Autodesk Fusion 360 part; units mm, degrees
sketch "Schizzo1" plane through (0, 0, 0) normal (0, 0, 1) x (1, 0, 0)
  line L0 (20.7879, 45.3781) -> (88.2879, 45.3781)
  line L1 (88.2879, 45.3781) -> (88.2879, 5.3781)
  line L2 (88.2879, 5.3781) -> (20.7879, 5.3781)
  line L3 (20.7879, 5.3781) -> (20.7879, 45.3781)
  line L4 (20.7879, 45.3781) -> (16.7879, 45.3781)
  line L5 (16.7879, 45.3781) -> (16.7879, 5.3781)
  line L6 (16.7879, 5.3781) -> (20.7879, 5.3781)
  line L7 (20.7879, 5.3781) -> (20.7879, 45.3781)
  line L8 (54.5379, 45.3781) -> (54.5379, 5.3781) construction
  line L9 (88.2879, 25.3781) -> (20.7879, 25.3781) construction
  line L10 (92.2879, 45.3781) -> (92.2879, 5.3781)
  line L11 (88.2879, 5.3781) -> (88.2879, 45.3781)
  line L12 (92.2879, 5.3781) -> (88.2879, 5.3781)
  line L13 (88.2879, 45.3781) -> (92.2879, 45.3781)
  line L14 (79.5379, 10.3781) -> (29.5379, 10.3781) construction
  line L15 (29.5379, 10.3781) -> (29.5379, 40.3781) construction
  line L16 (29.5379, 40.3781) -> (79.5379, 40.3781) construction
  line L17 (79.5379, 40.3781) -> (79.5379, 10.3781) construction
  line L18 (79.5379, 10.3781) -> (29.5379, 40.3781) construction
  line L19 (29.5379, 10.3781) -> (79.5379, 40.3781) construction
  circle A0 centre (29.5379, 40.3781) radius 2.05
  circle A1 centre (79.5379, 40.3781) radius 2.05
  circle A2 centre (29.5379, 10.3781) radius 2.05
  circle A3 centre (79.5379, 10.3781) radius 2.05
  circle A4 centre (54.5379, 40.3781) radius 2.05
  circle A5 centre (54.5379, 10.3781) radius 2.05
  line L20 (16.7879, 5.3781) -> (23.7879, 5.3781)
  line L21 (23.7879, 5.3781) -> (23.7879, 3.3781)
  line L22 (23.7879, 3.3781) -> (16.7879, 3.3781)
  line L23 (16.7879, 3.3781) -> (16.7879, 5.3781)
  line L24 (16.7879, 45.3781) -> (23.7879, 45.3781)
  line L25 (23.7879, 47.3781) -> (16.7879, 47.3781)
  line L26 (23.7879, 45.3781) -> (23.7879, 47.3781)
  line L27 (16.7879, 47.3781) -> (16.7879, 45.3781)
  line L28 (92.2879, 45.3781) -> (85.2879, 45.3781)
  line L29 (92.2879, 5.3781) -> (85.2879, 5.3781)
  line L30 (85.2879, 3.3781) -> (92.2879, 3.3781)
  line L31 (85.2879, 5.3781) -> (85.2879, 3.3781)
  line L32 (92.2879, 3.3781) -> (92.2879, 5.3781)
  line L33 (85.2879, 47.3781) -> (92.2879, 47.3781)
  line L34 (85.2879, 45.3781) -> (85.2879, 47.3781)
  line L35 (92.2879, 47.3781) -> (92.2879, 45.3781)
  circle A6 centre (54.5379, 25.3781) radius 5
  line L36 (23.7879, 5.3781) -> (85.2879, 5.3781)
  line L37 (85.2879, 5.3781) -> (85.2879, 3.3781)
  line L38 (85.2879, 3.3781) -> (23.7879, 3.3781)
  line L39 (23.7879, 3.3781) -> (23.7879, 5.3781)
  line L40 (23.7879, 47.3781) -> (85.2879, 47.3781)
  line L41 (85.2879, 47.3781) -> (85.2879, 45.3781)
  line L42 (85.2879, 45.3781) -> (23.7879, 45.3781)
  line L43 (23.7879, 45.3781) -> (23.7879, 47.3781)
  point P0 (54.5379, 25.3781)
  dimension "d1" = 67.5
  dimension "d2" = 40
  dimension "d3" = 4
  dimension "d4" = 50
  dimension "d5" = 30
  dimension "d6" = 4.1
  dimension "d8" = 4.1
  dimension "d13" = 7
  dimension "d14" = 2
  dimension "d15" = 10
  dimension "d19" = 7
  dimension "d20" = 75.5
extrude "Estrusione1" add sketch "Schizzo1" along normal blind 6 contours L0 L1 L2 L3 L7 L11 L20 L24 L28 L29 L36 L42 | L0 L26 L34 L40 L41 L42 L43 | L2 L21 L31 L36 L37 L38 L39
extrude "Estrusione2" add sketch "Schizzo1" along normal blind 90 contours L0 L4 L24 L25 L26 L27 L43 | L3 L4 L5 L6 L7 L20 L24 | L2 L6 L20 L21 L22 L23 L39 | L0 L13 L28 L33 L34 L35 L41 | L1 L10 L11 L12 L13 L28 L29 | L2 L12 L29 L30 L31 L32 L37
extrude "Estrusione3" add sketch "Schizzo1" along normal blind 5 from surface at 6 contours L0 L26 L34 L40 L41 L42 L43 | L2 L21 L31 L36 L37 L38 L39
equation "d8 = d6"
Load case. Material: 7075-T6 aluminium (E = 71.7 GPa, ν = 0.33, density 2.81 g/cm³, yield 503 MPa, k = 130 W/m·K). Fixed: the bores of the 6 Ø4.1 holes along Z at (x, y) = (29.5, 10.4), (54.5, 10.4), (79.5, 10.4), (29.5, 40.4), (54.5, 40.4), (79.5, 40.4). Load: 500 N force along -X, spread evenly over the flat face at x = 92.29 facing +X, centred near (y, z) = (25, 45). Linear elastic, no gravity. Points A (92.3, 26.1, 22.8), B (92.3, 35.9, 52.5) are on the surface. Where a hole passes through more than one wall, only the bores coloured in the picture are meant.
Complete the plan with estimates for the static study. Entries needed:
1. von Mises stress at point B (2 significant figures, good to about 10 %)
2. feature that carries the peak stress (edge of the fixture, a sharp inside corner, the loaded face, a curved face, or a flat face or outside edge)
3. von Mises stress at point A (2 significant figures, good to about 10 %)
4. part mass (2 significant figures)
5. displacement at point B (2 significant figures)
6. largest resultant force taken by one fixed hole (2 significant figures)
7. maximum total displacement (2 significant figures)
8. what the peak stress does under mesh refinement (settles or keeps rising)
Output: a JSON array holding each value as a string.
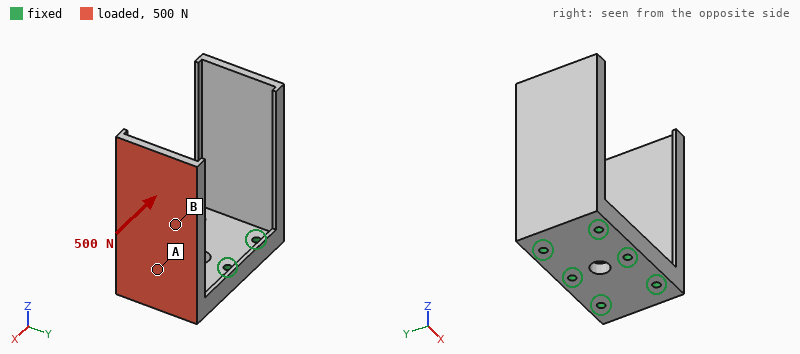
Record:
["25 MPa", "a sharp inside corner", "61 MPa", "150 g", "0.65 mm", "270 N", "1.5 mm", "keeps rising"]
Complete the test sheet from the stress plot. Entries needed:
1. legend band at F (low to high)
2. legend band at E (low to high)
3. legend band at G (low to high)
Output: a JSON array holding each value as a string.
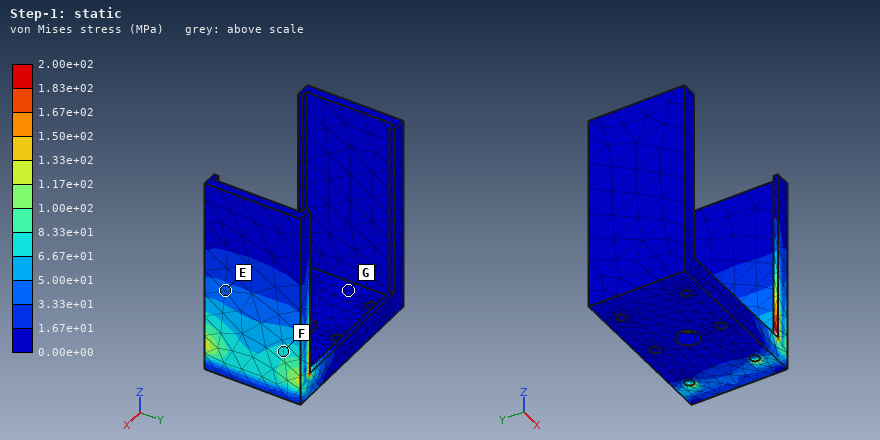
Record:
["6.67e+01 to 8.33e+01 MPa", "3.33e+01 to 5.00e+01 MPa", "0.00e+00 to 1.67e+01 MPa"]
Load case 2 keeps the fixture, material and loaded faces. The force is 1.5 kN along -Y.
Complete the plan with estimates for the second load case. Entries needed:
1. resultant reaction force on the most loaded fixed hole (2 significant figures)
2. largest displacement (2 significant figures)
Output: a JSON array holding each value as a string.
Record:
["2.2 kN", "0.19 mm"]
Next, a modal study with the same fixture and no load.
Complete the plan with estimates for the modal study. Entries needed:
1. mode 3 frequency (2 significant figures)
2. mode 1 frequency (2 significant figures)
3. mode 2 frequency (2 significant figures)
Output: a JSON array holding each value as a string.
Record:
["1800 Hz", "530 Hz", "530 Hz"]
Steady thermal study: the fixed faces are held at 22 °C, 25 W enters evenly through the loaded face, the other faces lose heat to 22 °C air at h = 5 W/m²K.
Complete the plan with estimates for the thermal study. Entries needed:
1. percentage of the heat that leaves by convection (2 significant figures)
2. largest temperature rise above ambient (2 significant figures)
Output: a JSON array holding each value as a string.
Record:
["4.0 %", "47 K"]
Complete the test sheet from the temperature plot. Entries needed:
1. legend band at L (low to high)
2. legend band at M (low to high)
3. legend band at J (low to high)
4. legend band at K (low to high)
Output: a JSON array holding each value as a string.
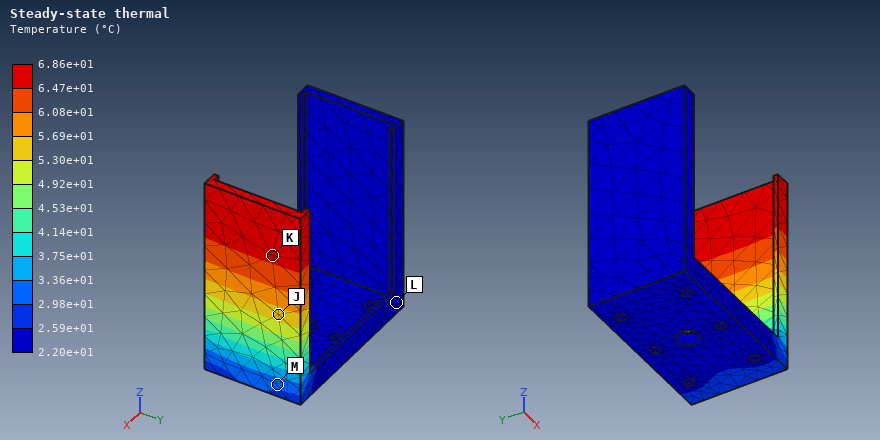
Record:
["2.20e+01 to 2.59e+01 °C", "2.98e+01 to 3.36e+01 °C", "5.30e+01 to 5.69e+01 °C", "6.47e+01 to 6.86e+01 °C"]
